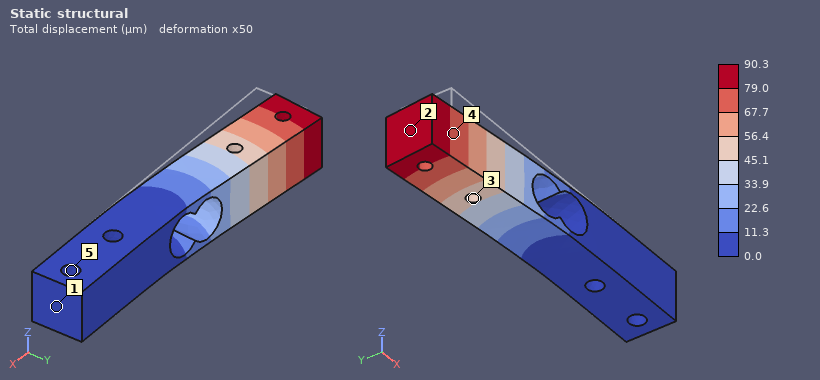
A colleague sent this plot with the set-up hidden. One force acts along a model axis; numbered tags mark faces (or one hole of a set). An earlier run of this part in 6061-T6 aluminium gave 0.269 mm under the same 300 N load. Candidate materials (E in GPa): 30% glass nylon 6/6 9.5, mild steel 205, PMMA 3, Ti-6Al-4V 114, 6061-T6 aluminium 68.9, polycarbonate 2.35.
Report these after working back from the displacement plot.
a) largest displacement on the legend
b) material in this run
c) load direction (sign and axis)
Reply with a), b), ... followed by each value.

a) 90.3 µm
b) mild steel
c) +Y
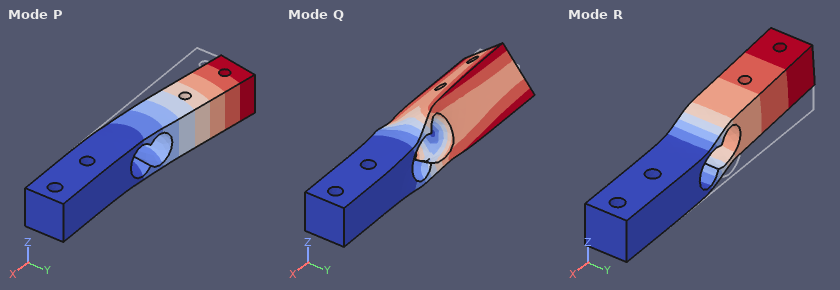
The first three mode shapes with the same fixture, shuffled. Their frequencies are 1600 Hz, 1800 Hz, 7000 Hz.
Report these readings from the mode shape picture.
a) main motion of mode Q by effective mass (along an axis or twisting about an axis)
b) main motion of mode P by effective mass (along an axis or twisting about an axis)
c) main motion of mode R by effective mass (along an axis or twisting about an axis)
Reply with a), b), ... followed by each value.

a) twisting about X
b) along Y
c) along Z
